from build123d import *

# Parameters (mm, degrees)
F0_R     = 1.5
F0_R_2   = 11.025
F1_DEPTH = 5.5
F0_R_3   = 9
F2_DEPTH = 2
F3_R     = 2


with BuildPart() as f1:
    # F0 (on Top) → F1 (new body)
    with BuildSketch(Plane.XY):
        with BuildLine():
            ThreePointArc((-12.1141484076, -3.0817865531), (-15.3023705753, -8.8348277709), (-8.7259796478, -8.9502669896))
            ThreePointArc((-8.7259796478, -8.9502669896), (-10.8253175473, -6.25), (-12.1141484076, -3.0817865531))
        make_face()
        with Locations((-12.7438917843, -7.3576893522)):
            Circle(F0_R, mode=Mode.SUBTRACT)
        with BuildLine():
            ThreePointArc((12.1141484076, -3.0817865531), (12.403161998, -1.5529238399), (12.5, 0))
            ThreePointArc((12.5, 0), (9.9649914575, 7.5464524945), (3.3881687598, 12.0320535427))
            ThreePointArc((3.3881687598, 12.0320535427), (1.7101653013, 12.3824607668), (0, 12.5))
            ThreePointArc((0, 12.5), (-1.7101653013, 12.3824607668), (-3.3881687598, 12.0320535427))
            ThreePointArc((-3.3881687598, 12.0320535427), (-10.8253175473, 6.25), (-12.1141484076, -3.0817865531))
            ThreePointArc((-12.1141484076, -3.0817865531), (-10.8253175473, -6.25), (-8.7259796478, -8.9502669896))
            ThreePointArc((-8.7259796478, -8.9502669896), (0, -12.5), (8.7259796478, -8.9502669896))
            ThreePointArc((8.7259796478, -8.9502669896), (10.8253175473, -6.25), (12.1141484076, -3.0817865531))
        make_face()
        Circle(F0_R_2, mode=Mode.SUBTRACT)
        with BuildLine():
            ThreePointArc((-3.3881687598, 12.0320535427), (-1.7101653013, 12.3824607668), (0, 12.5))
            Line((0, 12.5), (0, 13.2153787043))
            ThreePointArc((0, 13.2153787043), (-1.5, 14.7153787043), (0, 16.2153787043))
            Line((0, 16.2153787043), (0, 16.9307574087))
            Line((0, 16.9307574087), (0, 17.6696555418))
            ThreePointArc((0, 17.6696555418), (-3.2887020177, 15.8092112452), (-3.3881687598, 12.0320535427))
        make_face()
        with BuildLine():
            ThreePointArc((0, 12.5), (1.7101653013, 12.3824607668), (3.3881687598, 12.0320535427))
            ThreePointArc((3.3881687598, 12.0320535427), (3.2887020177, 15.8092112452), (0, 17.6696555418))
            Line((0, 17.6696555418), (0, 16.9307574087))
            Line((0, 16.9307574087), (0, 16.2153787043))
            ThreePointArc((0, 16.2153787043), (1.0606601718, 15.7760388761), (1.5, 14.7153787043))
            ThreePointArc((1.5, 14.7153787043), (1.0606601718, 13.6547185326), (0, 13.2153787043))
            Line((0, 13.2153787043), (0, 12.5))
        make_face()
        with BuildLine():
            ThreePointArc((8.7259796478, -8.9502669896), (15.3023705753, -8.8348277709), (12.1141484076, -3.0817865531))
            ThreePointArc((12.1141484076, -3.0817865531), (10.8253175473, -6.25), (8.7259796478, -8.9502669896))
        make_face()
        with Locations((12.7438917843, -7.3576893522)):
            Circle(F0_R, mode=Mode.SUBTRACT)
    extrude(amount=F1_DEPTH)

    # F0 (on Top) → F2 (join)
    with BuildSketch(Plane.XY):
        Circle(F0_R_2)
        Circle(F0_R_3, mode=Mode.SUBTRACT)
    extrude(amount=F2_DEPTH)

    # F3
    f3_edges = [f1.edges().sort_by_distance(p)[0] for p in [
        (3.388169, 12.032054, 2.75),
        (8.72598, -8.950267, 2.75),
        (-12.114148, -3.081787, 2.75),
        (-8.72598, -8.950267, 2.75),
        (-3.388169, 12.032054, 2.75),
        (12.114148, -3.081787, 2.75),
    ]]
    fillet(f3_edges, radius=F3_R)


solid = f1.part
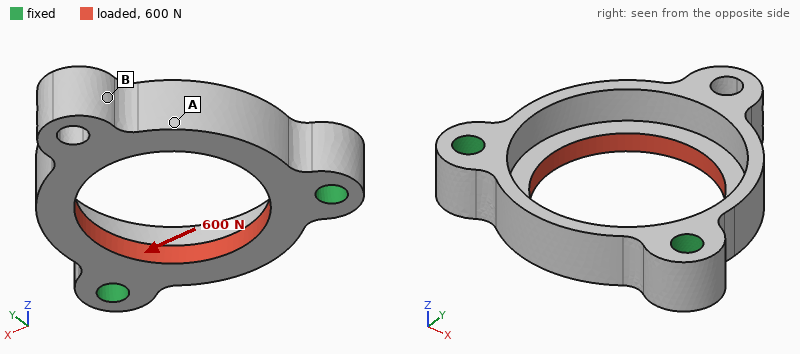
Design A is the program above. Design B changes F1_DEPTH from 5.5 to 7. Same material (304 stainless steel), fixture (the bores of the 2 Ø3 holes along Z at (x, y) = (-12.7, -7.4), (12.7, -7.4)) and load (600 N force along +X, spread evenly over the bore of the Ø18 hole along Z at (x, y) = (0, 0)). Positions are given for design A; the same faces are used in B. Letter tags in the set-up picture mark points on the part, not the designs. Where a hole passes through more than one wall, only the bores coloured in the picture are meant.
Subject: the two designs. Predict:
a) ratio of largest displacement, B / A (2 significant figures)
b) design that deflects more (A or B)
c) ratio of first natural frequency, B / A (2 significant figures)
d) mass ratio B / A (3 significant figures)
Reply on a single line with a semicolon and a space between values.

0.91; A; 1.2; 1.22
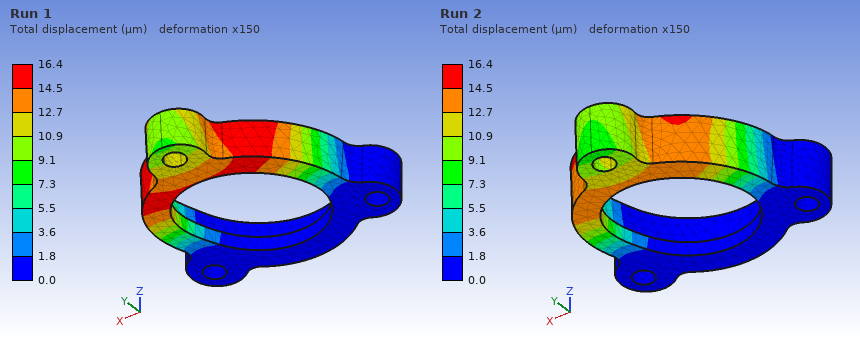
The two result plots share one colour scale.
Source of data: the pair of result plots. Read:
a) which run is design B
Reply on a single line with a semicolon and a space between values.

Run 2
